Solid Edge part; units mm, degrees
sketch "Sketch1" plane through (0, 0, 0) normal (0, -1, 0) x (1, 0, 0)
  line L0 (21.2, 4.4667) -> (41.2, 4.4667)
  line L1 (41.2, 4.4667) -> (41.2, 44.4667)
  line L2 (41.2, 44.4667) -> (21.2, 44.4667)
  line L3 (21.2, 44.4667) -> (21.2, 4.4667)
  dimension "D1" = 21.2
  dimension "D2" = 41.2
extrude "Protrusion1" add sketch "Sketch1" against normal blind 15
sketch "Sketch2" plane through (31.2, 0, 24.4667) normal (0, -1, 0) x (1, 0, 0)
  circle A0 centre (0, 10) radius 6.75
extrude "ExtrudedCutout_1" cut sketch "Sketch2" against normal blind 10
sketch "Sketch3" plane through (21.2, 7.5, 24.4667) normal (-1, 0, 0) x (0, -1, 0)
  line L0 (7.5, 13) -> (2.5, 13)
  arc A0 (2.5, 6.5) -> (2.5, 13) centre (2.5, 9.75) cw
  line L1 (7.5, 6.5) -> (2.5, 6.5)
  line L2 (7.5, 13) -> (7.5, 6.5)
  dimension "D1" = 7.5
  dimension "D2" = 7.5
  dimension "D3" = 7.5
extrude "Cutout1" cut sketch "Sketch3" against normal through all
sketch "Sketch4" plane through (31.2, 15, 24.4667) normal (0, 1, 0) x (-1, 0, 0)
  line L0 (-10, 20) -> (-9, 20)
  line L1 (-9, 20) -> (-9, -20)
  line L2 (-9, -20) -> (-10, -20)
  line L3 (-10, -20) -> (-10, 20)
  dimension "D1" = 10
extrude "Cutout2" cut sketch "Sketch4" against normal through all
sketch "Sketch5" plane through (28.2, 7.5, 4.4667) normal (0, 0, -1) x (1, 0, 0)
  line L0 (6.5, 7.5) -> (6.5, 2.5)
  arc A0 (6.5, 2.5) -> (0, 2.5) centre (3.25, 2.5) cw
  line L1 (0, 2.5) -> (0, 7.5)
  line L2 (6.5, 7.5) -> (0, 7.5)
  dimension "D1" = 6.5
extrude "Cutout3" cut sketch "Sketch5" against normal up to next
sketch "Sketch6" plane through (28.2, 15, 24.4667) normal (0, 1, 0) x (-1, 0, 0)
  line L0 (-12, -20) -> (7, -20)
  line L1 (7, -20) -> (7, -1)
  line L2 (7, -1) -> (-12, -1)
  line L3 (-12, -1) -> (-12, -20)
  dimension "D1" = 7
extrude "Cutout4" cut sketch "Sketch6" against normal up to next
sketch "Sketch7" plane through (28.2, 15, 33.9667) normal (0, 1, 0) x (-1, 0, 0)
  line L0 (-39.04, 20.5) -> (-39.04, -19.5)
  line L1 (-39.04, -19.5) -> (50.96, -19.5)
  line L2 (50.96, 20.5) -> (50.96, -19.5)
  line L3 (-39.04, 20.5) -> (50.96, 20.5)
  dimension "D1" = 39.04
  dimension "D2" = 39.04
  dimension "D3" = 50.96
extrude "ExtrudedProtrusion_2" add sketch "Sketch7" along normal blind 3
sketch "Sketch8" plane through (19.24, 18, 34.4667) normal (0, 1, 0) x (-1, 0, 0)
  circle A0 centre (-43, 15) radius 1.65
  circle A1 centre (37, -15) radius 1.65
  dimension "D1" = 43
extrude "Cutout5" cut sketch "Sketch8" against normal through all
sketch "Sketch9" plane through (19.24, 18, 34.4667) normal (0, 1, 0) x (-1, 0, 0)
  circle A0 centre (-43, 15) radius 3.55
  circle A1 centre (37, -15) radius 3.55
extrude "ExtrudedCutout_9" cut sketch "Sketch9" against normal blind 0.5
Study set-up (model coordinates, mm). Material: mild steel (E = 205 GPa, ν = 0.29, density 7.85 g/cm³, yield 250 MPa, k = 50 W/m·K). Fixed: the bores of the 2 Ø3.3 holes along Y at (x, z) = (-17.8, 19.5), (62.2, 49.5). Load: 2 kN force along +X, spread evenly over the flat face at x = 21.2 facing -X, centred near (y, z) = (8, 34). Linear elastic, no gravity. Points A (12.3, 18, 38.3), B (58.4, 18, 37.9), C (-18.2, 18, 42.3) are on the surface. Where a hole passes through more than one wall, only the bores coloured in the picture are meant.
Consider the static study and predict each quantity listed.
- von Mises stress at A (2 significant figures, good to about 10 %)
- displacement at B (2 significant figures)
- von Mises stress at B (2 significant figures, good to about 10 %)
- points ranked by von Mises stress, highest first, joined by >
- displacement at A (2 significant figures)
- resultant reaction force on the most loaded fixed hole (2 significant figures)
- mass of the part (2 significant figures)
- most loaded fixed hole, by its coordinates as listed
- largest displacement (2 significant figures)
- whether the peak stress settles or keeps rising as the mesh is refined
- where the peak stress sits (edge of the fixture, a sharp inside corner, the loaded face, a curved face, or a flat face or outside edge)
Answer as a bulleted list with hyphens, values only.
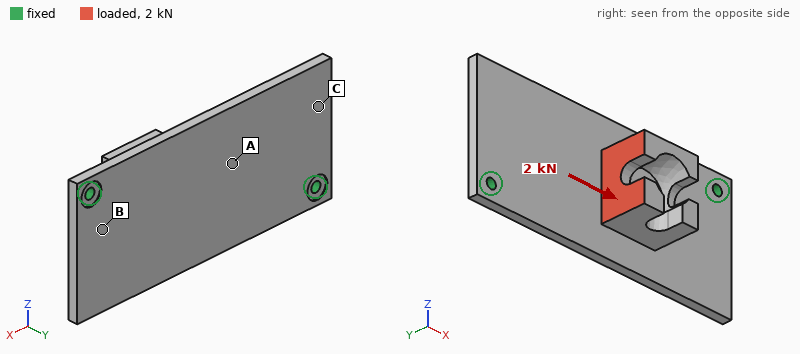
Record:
- 70 MPa
- 0.033 mm
- 38 MPa
- A > B > C
- 0.095 mm
- 1.1 kN
- 120 g
- (62.2, 49.5)
- 0.16 mm
- keeps rising
- edge of the fixture
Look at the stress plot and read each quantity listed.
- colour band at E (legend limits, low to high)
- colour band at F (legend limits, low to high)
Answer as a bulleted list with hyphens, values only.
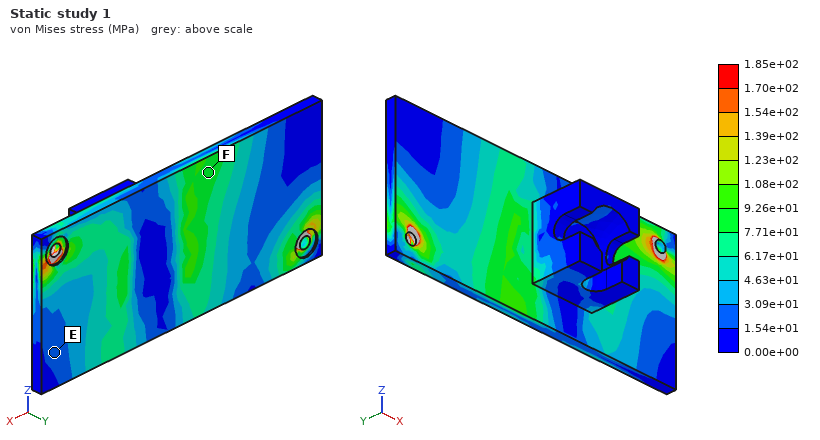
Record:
- 1.54e+01 to 3.09e+01 MPa
- 7.71e+01 to 9.26e+01 MPa
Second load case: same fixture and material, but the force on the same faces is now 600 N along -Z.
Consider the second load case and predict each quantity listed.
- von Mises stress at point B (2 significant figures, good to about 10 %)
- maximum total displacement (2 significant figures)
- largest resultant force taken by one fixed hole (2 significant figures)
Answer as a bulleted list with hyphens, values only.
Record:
- 36 MPa
- 0.11 mm
- 300 N
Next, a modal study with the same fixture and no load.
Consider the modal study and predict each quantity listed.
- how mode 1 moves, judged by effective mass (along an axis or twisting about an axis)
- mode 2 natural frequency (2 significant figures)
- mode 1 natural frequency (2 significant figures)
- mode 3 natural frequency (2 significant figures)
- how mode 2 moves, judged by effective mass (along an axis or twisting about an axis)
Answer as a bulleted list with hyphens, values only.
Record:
- along Y
- 1400 Hz
- 1300 Hz
- 3400 Hz
- along Y
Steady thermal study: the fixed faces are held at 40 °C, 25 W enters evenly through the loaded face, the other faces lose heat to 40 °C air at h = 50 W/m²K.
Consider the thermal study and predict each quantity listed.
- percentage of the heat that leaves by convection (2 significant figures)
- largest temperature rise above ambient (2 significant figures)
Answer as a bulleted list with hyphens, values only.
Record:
- 64 %
- 81 K
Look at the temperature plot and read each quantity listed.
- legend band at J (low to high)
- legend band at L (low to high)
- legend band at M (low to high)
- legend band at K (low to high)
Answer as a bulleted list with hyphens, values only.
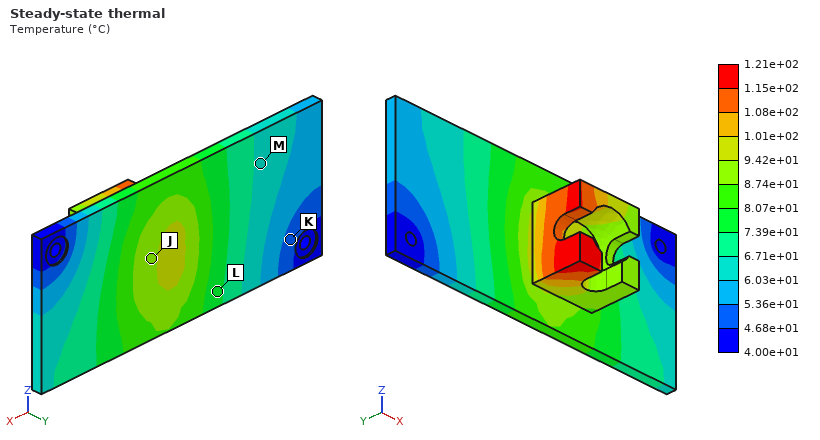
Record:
- 8.74e+01 to 9.42e+01 °C
- 7.39e+01 to 8.07e+01 °C
- 6.03e+01 to 6.71e+01 °C
- 4.68e+01 to 5.36e+01 °C
